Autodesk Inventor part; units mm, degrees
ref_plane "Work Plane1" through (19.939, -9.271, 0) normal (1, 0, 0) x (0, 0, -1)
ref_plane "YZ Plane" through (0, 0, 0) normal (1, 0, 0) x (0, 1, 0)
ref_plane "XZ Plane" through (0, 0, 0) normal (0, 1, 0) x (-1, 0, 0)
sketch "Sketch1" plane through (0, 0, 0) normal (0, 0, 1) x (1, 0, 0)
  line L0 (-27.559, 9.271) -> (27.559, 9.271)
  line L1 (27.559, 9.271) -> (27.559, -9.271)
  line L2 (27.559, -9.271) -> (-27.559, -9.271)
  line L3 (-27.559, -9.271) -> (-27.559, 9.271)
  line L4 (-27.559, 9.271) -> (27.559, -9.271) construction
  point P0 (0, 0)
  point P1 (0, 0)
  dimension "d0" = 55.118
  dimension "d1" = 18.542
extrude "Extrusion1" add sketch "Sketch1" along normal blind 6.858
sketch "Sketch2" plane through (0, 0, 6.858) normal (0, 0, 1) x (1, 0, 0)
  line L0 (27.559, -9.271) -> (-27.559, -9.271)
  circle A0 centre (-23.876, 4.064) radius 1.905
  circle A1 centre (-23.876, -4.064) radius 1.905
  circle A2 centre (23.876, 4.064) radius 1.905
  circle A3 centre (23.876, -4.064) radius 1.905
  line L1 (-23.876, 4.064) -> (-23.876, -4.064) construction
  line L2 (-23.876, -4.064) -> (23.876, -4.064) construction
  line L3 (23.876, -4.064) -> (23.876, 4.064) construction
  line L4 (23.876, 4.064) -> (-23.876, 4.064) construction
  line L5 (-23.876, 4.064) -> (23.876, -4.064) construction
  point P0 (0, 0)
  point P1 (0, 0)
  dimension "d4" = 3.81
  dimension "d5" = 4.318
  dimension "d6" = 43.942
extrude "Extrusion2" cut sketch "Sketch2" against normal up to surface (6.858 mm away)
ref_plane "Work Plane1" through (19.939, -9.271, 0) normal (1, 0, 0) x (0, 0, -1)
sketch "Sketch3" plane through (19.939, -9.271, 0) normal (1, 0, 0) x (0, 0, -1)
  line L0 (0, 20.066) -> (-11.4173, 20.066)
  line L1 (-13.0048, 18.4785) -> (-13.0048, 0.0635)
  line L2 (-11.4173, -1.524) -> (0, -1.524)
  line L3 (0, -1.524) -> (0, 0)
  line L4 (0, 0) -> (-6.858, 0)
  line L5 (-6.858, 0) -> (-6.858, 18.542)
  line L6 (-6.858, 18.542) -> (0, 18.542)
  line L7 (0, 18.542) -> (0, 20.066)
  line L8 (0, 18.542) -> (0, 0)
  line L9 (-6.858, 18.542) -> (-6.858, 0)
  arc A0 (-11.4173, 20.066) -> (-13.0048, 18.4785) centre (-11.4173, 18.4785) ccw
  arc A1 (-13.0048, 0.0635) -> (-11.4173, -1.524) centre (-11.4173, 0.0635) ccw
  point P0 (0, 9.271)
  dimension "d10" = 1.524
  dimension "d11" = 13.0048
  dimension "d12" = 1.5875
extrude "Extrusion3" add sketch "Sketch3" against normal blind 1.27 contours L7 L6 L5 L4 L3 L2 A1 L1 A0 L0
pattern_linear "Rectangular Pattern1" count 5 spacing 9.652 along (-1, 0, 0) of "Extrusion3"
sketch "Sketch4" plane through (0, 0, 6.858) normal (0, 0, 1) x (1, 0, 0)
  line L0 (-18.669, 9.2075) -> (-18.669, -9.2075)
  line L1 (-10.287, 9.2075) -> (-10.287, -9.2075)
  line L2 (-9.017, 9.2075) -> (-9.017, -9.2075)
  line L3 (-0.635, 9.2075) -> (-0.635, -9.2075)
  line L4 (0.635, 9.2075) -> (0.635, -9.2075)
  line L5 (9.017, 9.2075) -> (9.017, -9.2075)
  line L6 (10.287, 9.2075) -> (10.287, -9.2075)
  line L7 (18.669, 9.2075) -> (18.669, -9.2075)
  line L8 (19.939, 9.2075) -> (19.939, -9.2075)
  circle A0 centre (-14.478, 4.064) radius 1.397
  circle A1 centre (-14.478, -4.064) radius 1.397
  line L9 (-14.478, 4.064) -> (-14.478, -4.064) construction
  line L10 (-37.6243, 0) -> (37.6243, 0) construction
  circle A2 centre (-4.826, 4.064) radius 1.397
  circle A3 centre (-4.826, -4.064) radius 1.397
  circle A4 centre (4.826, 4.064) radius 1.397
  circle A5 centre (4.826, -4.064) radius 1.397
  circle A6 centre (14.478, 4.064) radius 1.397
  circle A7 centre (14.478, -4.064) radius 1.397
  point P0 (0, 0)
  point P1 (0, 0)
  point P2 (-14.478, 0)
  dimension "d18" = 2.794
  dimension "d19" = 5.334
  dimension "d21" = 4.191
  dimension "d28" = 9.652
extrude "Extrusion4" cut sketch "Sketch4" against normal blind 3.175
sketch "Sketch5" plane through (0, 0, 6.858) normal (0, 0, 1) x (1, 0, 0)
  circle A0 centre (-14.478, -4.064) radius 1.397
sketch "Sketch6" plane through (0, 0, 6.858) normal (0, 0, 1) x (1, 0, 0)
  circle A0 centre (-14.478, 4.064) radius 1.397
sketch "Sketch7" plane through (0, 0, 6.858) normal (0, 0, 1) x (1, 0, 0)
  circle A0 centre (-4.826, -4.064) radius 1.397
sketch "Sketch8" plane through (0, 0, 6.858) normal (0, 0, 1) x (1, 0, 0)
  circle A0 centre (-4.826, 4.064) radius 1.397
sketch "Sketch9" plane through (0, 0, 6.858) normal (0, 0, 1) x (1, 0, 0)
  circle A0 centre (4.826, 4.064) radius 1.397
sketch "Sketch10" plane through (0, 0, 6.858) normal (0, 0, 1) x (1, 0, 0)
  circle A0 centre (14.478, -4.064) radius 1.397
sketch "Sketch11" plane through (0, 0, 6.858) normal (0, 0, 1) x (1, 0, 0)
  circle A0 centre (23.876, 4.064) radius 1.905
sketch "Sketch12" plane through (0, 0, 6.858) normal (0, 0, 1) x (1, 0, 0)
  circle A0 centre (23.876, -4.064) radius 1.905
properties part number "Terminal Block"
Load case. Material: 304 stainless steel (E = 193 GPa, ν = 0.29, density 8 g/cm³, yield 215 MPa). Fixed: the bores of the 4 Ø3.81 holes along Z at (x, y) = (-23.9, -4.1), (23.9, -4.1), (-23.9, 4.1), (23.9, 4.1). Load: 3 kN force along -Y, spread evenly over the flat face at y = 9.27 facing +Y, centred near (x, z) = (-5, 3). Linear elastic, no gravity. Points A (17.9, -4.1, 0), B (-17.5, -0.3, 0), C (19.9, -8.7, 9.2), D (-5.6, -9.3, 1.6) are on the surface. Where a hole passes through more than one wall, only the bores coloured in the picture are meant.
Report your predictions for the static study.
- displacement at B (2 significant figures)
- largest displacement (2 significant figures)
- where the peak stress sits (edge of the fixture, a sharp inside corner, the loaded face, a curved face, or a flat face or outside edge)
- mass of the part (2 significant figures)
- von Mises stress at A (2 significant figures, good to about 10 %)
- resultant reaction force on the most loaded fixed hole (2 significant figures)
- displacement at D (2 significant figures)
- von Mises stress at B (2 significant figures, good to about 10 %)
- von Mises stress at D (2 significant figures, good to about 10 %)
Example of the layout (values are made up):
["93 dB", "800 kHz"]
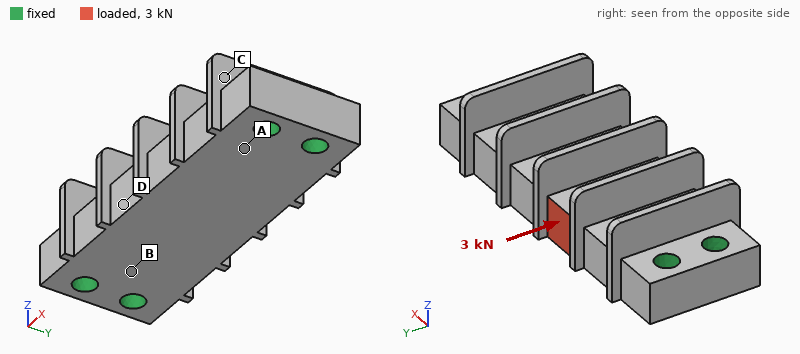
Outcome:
["1.8 µm", "8.2 µm", "a curved face", "60 g", "23 MPa", "1.7 kN", "5.3 µm", "44 MPa", "36 MPa"]
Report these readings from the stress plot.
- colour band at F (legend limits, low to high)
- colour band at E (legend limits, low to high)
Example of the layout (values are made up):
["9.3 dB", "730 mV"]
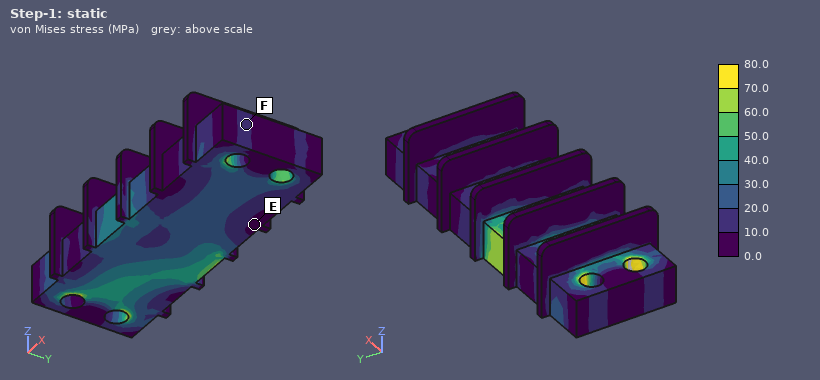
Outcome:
["10.0 to 20.0 MPa", "0.0 to 10.0 MPa"]
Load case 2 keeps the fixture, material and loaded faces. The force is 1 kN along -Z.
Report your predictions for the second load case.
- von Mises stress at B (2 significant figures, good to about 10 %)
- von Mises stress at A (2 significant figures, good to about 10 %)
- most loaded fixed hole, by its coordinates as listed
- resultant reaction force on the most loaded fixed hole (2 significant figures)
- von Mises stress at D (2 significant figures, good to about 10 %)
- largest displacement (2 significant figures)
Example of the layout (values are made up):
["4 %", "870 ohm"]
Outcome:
["36 MPa", "22 MPa", "(-23.9, 4.1)", "690 N", "7.7 MPa", "15 µm"]
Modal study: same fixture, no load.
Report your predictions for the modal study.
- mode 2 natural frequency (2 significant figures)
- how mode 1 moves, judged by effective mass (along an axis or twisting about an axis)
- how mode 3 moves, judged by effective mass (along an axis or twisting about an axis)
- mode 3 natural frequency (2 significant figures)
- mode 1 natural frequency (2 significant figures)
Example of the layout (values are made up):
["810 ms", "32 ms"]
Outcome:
["18 kHz", "along Z", "along Y", "22 kHz", "13 kHz"]
